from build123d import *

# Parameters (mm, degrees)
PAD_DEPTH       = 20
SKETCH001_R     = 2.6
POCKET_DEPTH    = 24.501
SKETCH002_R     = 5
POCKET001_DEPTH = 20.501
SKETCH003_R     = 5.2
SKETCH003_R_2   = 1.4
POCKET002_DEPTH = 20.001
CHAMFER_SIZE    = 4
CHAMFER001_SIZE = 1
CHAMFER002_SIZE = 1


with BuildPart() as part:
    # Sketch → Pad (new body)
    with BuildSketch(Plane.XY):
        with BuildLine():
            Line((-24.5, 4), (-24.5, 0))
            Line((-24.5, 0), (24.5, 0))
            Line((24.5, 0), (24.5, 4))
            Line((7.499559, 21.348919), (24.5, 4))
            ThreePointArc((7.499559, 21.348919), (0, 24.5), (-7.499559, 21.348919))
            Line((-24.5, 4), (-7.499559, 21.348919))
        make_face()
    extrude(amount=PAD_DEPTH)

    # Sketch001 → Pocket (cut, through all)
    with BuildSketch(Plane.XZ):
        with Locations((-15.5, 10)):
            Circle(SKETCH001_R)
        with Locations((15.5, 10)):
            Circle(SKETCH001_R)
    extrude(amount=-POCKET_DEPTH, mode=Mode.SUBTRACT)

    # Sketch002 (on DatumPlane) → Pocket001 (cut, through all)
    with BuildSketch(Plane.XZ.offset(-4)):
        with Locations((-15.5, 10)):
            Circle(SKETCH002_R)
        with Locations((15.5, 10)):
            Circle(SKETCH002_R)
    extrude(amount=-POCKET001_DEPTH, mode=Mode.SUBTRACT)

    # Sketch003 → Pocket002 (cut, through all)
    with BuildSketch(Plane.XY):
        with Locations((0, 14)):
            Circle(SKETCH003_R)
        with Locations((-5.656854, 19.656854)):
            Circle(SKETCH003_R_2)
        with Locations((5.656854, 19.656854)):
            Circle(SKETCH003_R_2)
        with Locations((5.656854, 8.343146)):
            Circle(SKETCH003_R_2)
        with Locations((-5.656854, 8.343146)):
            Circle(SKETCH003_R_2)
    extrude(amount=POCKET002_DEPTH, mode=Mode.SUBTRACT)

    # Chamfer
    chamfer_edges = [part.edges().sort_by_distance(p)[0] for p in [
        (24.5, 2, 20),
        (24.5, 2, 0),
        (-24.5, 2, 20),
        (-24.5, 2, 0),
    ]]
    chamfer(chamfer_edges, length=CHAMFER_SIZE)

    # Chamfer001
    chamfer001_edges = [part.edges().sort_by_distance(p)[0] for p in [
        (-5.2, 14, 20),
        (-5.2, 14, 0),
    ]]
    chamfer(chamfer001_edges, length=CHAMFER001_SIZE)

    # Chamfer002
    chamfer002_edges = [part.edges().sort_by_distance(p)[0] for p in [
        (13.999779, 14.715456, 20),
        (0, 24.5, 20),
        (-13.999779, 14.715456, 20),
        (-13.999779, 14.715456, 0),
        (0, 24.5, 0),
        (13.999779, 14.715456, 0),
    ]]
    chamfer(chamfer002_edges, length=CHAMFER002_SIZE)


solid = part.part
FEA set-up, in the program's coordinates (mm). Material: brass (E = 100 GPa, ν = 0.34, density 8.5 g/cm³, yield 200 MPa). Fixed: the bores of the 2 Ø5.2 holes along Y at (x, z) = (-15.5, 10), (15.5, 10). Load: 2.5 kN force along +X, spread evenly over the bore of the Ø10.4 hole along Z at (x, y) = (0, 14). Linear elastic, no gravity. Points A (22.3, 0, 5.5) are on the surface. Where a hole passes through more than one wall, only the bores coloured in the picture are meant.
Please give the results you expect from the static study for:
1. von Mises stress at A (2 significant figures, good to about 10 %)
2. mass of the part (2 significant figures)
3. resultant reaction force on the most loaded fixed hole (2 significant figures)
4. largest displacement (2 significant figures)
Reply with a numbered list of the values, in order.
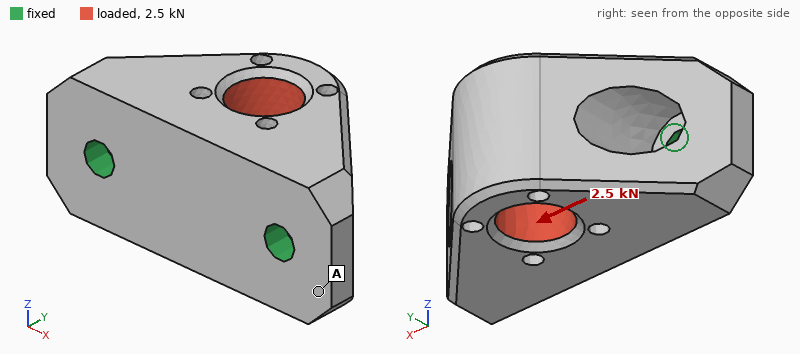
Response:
1. 10.0 MPa
2. 99 g
3. 1.6 kN
4. 6.5 µm
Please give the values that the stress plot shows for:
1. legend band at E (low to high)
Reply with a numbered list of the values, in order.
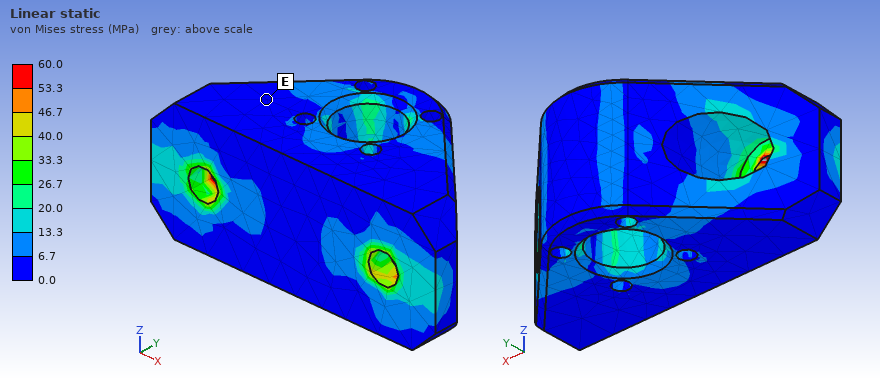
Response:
1. 0.0 to 6.7 MPa
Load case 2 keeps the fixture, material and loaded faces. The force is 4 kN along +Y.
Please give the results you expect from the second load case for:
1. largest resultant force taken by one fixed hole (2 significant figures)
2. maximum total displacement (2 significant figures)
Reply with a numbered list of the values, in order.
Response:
1. 2.2 kN
2. 7.4 µm
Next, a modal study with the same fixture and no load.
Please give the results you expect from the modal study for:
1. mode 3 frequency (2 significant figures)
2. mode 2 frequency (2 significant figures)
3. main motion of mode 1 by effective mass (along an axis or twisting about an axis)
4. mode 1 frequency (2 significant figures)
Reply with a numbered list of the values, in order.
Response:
1. 15 kHz
2. 15 kHz
3. along Z
4. 5500 Hz
